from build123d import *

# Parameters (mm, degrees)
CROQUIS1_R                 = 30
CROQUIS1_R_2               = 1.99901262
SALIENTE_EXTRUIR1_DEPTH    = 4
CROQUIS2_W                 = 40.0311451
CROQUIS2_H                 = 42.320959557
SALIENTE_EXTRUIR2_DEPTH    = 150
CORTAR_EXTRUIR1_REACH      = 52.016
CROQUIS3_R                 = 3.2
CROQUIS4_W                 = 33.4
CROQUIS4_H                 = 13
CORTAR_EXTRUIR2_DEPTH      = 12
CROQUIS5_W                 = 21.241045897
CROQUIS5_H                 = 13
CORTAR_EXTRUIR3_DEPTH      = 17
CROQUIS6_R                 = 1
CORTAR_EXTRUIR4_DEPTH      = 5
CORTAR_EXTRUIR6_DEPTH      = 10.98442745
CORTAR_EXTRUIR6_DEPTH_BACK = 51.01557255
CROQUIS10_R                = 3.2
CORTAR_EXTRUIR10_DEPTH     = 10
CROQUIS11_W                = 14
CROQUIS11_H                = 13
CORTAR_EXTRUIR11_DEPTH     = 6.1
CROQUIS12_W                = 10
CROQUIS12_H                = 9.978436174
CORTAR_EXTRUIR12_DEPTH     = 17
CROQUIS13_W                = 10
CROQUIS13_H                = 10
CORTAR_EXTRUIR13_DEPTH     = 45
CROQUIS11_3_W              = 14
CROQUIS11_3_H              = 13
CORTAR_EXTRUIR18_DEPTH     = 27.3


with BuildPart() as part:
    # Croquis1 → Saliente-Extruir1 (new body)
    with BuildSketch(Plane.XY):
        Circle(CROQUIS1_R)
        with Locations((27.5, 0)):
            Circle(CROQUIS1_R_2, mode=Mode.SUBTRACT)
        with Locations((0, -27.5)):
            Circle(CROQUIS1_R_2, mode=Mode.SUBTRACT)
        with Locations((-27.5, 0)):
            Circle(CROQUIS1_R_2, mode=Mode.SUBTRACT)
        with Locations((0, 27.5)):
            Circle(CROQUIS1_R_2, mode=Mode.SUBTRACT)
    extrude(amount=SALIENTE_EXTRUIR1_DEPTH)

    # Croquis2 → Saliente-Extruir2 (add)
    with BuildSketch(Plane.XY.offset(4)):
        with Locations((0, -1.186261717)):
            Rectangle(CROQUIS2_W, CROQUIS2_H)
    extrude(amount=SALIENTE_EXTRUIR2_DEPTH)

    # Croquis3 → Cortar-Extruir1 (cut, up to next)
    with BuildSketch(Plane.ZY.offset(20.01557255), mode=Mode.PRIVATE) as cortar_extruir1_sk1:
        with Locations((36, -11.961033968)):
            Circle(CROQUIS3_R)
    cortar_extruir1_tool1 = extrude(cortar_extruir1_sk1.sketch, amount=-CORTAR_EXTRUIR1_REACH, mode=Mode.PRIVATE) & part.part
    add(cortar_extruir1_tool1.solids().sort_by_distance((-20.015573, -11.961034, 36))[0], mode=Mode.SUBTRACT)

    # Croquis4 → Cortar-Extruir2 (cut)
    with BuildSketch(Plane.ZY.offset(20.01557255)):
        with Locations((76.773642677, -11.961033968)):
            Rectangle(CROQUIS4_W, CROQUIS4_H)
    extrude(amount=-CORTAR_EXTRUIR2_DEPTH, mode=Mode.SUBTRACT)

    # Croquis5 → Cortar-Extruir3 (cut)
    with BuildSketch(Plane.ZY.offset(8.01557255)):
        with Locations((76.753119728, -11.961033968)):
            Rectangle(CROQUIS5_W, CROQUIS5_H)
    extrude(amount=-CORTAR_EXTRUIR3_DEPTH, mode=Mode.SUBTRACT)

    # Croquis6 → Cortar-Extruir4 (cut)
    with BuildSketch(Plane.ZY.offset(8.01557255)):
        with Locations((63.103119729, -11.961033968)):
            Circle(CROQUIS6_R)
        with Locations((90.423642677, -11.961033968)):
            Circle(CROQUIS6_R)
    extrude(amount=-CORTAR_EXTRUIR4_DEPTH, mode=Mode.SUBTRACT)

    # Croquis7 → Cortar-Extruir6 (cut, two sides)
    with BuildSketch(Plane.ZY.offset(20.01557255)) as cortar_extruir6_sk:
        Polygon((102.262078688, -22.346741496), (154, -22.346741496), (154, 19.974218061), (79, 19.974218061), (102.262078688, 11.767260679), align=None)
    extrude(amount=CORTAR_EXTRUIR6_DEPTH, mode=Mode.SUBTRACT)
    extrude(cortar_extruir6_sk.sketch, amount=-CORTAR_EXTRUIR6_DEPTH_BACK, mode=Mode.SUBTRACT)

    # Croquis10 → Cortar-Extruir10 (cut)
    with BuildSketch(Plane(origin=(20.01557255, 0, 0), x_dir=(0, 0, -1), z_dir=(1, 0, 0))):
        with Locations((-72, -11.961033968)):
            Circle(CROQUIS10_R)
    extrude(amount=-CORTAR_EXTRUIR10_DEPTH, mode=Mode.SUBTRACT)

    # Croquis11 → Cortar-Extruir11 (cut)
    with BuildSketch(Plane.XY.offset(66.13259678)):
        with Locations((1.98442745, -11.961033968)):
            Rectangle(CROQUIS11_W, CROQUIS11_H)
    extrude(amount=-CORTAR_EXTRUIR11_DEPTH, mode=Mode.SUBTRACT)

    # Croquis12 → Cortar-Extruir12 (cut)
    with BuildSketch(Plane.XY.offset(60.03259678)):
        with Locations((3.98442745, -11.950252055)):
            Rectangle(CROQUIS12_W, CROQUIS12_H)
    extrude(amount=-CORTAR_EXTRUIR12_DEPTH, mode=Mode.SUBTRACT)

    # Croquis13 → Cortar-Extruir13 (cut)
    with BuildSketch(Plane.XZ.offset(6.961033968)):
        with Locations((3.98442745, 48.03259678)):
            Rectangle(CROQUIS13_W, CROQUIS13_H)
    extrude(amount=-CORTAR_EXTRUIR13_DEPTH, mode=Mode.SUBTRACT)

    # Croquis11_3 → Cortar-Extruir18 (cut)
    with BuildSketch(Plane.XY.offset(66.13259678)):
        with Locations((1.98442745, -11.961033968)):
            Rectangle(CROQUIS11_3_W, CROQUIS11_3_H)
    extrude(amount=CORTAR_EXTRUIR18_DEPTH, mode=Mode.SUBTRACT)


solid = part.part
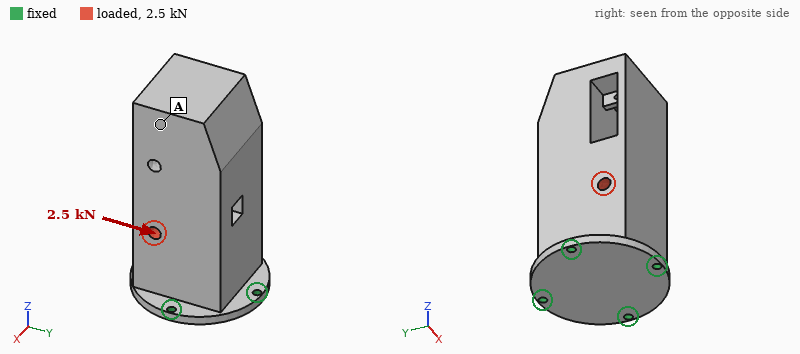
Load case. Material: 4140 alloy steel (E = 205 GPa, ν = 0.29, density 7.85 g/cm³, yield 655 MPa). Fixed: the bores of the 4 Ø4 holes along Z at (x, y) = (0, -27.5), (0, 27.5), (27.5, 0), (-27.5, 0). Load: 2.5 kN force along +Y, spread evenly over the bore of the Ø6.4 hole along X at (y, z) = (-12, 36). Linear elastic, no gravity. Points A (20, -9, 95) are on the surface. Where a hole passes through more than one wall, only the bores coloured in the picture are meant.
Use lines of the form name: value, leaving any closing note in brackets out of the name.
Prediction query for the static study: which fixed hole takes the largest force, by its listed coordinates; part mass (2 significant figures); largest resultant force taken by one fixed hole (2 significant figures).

which fixed hole takes the largest force, by its listed coordinates: (0, -27.5)
part mass: 1.2 kg
largest resultant force taken by one fixed hole: 2.2 kN
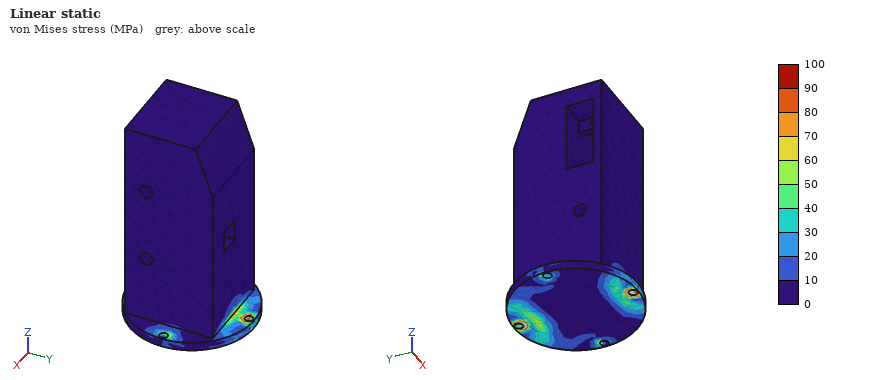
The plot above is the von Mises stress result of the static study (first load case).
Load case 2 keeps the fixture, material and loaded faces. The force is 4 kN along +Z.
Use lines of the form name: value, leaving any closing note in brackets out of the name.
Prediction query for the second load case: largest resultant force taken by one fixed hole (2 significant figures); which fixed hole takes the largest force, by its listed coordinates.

largest resultant force taken by one fixed hole: 2.2 kN
which fixed hole takes the largest force, by its listed coordinates: (0, -27.5)
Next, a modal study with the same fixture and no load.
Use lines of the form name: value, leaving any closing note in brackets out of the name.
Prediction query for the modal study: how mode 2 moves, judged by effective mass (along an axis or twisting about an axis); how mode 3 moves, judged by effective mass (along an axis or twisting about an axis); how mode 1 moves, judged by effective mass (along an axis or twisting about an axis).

how mode 2 moves, judged by effective mass: along Y
how mode 3 moves, judged by effective mass: along Z
how mode 1 moves, judged by effective mass: along X
